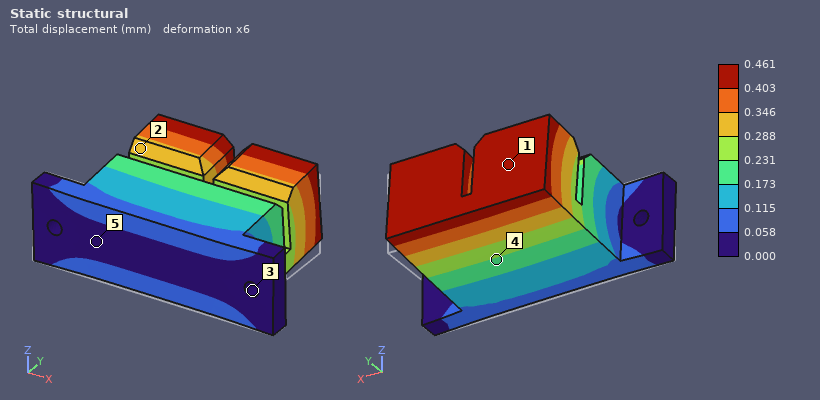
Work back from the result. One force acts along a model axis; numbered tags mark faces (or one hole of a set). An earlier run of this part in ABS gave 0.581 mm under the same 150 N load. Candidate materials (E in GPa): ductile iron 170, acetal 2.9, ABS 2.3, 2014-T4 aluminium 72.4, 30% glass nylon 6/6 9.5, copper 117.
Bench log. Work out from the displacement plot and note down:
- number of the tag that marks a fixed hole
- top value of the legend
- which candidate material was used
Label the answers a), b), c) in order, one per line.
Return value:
a) 3
b) 0.461 mm
c) acetal
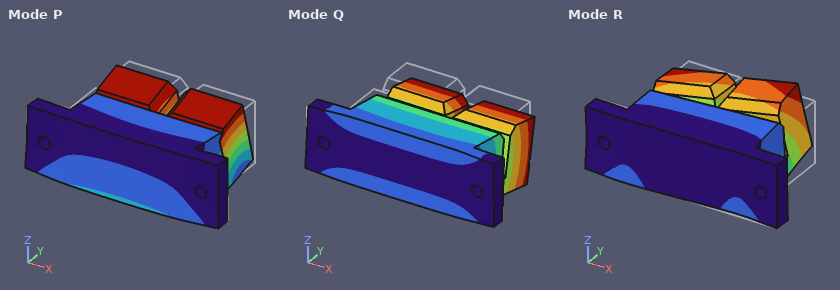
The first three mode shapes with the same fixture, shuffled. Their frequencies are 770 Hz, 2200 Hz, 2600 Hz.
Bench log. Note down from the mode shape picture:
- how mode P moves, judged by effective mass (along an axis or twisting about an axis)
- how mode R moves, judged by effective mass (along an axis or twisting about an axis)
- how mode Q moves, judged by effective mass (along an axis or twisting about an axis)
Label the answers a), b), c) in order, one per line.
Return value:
a) along Y
b) along X
c) along Z
